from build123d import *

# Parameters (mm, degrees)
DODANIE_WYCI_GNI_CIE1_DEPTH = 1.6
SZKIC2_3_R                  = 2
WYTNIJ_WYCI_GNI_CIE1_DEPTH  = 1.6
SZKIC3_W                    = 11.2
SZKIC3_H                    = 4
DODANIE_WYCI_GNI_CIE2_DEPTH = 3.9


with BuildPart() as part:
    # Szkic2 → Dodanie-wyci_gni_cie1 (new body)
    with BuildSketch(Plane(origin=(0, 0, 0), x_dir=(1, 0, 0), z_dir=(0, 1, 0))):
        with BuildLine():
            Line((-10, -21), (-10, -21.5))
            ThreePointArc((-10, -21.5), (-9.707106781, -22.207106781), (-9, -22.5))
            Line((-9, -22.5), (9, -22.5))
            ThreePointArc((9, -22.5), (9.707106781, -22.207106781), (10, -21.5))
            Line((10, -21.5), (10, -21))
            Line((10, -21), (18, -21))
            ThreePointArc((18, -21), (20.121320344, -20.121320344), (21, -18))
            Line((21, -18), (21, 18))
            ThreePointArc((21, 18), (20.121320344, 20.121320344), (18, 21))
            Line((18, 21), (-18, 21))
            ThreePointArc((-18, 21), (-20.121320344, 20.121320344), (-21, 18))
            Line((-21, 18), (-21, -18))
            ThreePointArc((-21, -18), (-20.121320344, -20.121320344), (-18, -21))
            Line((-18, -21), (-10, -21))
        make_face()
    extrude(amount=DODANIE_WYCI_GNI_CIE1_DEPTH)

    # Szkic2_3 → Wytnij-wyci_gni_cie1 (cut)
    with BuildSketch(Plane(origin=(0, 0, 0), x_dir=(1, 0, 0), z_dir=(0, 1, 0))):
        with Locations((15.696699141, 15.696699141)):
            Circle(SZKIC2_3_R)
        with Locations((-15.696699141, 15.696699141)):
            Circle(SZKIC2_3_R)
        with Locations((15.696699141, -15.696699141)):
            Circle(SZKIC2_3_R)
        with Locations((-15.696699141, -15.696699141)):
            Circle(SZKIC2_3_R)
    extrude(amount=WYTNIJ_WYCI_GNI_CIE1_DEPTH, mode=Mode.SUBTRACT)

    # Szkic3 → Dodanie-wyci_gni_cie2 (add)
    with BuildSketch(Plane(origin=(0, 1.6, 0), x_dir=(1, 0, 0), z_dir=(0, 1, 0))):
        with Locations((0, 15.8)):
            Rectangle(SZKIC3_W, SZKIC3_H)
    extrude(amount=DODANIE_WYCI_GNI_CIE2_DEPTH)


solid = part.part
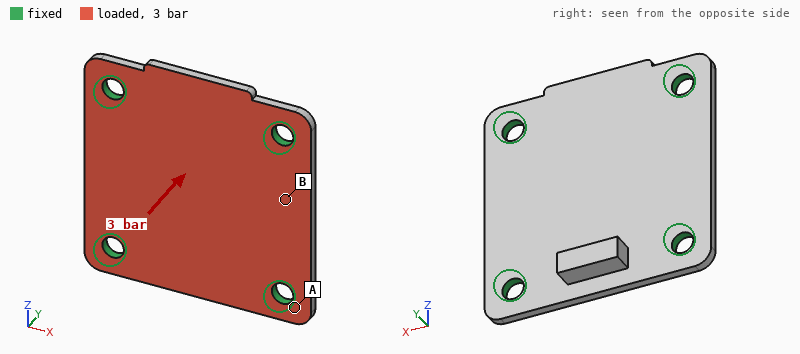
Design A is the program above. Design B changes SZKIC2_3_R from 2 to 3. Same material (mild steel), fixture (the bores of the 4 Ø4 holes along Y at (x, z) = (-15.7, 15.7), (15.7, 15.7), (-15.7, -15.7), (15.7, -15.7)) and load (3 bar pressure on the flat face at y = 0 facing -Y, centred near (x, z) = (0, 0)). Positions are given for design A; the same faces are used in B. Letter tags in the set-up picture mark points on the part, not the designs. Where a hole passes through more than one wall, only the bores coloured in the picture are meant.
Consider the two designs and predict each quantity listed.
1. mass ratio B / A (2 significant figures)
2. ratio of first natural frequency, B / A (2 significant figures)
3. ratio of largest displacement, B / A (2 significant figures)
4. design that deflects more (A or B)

0.97
1.1
0.77
A
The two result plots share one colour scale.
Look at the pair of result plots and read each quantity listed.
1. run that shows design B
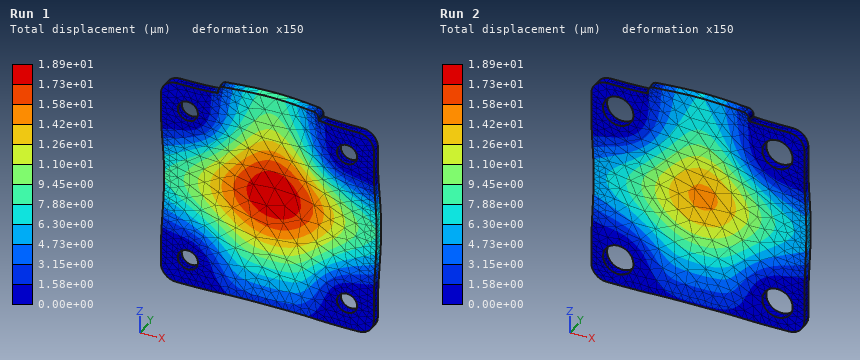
Run 2
